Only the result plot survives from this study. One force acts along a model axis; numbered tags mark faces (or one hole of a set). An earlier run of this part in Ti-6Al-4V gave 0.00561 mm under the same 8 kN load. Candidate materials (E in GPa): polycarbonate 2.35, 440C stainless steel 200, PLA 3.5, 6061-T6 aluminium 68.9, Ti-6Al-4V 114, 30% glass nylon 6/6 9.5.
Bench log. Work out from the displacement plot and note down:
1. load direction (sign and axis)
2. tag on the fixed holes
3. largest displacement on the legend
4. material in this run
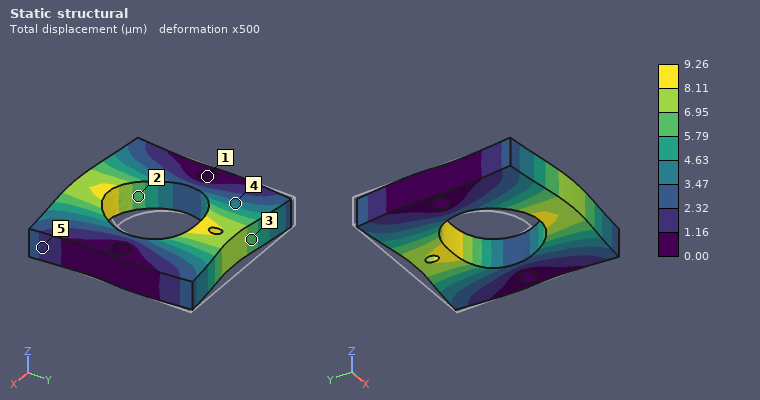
-Y
1
9.26 µm
6061-T6 aluminium
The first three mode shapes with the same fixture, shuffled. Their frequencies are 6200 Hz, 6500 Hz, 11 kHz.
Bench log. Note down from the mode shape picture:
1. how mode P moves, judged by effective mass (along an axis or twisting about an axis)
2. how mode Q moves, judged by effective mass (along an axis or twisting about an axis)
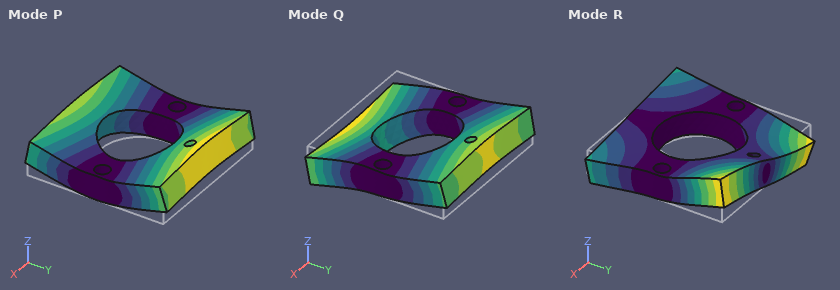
along Z
twisting about X
